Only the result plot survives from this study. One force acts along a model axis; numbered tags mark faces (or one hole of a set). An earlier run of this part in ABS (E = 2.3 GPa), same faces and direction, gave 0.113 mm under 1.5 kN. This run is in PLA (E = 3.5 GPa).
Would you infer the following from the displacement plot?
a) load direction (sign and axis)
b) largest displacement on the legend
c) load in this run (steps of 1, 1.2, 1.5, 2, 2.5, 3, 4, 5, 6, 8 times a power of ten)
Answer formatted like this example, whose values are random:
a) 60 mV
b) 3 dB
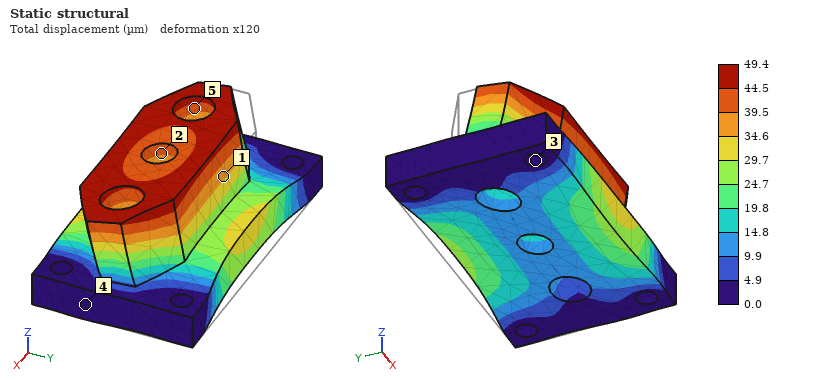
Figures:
a) -Y
b) 49.4 µm
c) 1 kN
